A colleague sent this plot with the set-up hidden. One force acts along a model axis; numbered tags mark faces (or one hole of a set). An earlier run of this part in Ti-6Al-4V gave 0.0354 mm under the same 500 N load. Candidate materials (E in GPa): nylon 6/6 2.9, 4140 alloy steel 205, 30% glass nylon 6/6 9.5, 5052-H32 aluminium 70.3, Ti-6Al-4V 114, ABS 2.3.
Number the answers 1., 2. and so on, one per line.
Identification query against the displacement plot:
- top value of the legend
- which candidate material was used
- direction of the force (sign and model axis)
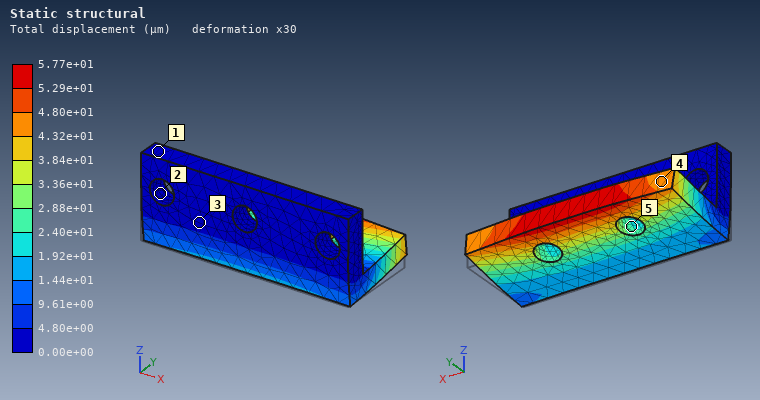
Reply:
1. 5.77e+01 µm
2. 5052-H32 aluminium
3. +Z
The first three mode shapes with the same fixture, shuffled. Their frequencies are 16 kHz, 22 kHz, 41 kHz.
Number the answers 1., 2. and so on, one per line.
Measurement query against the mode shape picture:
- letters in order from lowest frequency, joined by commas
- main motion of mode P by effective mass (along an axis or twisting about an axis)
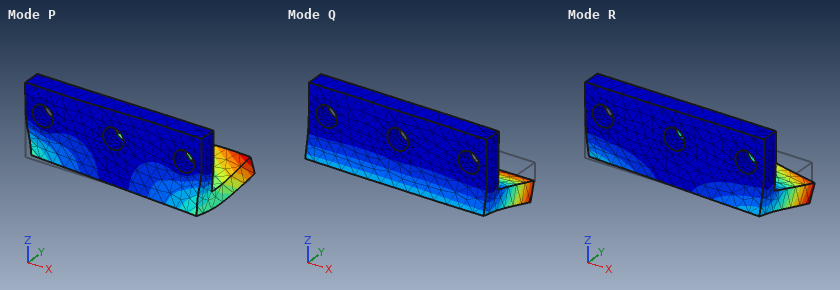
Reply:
1. Q, R, P
2. along X
